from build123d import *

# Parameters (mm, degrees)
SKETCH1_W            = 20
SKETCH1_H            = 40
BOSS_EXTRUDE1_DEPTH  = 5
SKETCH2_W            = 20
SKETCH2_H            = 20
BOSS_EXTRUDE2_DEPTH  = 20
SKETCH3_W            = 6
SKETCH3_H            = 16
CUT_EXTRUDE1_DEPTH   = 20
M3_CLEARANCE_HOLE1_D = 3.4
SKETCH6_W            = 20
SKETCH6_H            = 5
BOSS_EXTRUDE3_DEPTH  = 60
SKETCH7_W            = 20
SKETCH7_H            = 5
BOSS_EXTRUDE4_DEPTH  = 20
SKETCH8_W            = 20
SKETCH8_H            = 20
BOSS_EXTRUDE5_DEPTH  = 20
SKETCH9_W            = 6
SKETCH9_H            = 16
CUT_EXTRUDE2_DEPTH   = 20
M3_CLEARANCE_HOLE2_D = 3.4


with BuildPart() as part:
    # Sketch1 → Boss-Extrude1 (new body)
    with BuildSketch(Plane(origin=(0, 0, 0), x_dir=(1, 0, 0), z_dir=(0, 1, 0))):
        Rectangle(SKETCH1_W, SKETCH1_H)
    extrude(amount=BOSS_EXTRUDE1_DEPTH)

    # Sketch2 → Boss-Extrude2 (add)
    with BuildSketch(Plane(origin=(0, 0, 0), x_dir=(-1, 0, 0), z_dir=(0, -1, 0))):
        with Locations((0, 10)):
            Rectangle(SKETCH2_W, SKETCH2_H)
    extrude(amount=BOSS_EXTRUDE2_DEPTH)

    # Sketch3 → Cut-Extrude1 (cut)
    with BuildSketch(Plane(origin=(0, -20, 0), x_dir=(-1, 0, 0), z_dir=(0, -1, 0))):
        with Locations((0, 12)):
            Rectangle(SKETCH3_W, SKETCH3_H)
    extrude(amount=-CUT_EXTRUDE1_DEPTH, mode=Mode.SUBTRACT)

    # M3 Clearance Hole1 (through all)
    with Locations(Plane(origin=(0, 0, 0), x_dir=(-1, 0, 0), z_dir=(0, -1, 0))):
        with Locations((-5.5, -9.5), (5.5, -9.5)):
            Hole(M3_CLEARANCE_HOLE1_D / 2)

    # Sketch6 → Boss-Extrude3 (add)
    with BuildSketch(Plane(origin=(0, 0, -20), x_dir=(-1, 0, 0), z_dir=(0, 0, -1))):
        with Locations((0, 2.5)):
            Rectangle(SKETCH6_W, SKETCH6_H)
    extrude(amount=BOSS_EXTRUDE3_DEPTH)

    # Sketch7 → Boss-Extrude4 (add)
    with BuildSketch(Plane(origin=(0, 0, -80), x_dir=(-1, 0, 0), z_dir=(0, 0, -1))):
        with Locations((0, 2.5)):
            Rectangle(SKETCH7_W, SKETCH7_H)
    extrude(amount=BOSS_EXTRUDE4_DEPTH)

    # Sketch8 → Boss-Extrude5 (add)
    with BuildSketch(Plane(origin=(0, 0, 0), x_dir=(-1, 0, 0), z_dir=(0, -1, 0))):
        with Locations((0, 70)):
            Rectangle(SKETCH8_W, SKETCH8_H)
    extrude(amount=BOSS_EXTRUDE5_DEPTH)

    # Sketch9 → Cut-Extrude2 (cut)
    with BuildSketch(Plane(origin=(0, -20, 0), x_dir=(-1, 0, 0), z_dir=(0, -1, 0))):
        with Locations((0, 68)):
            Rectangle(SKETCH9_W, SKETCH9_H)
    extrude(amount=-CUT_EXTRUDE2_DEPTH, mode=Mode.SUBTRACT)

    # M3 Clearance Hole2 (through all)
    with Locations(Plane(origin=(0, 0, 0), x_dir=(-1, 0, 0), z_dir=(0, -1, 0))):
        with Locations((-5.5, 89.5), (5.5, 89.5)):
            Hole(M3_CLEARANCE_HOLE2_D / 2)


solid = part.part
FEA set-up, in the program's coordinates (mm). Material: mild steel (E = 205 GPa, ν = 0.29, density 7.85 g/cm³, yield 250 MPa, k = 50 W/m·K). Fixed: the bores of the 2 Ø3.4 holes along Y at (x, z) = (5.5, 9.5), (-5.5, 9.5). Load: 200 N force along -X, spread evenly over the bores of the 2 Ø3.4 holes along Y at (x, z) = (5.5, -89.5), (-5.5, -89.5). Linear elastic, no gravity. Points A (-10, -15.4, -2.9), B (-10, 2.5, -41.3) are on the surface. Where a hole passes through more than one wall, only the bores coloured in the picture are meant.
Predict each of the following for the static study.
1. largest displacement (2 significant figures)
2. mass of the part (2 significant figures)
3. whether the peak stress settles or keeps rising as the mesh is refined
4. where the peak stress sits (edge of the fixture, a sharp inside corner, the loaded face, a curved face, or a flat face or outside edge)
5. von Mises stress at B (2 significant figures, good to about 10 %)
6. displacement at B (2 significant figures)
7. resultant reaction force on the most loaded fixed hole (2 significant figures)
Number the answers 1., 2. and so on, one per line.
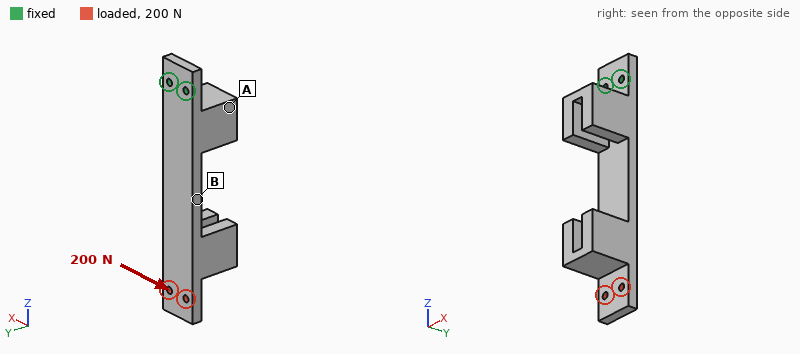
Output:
1. 0.10 mm
2. 190 g
3. keeps rising
4. edge of the fixture
5. 29 MPa
6. 0.031 mm
7. 1.6 kN
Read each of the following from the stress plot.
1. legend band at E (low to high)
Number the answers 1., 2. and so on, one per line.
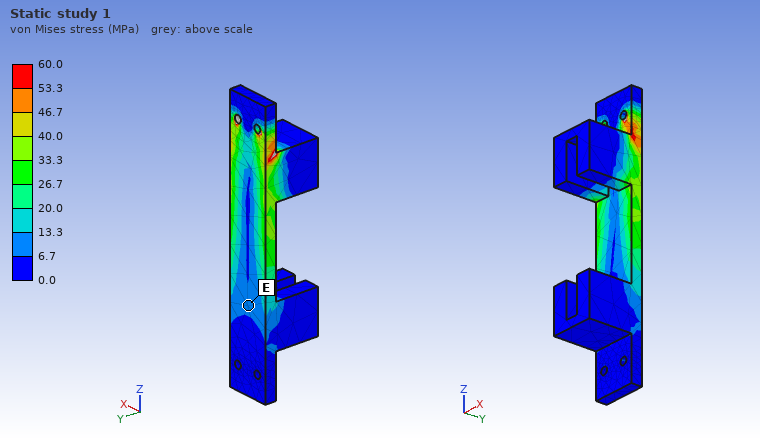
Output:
1. 6.7 to 13.3 MPa
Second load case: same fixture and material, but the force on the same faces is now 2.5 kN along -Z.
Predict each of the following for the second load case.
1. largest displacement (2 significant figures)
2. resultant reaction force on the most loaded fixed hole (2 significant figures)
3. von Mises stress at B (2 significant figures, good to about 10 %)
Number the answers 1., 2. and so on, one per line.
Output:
1. 35 µm
2. 1.3 kN
3. 25 MPa
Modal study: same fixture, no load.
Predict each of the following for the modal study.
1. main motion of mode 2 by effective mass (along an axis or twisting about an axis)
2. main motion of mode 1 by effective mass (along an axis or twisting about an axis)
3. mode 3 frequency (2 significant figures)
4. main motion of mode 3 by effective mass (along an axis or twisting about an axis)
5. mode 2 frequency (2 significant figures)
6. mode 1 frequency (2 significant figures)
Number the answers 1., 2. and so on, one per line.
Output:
1. along X
2. along Y
3. 1700 Hz
4. along Y
5. 950 Hz
6. 300 Hz
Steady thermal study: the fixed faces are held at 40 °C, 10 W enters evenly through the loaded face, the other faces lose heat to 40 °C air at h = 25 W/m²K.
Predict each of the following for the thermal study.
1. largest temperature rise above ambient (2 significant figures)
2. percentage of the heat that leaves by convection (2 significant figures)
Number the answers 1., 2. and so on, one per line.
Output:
1. 75 K
2. 75 %
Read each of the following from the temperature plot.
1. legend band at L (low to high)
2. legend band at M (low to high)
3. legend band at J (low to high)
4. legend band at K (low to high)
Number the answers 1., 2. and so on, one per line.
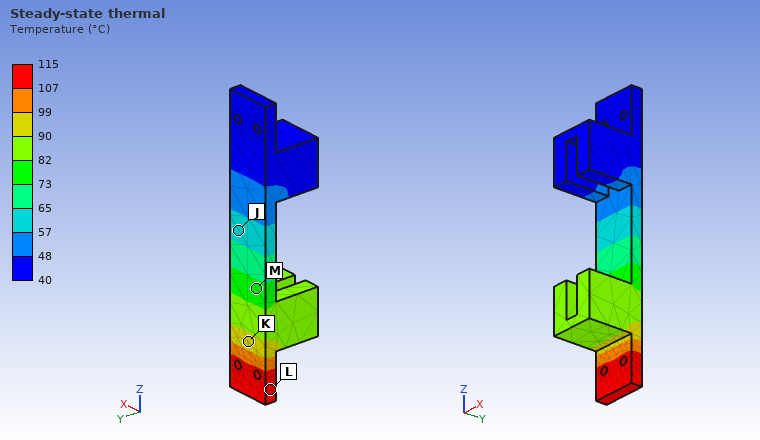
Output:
1. 107 to 115 °C
2. 73 to 82 °C
3. 57 to 65 °C
4. 90 to 99 °C
